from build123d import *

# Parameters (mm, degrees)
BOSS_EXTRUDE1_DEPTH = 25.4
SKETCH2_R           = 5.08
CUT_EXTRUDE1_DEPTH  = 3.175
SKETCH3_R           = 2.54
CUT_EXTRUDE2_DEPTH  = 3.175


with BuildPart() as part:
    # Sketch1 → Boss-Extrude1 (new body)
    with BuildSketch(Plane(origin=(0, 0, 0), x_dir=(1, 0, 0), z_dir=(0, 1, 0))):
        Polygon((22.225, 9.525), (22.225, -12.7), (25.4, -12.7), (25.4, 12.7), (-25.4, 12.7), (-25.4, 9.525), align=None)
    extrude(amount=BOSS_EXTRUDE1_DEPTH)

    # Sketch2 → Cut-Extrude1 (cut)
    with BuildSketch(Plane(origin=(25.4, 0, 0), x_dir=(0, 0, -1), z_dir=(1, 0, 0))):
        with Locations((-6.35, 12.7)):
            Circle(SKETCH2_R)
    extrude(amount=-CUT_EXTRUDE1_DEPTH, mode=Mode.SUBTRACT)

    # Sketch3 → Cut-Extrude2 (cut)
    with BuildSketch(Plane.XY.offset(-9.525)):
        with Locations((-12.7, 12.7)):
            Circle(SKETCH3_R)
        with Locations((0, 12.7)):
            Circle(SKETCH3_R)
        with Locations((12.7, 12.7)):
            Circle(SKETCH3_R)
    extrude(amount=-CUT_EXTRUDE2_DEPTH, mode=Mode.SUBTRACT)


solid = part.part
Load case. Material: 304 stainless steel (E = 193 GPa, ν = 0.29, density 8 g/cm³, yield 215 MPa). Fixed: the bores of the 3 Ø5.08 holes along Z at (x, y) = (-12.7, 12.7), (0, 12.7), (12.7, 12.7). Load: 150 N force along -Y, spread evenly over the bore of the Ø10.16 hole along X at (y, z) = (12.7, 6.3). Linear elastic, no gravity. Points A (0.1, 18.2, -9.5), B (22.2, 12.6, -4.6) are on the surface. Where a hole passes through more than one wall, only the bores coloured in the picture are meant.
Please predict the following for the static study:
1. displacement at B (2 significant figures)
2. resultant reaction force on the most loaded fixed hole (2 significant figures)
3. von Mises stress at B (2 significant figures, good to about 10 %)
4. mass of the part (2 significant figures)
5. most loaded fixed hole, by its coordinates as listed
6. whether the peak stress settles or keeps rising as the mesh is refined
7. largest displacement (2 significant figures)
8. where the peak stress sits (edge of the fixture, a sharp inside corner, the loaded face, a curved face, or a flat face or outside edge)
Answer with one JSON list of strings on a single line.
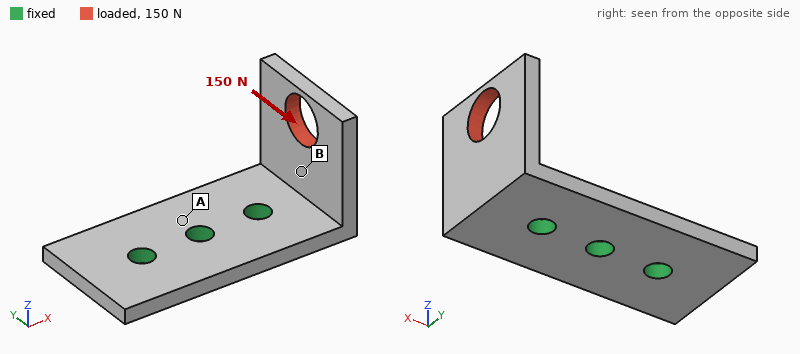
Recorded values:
["7.8 µm", "200 N", "16 MPa", "44 g", "(12.7, 12.7)", "keeps rising", "31 µm", "edge of the fixture"]
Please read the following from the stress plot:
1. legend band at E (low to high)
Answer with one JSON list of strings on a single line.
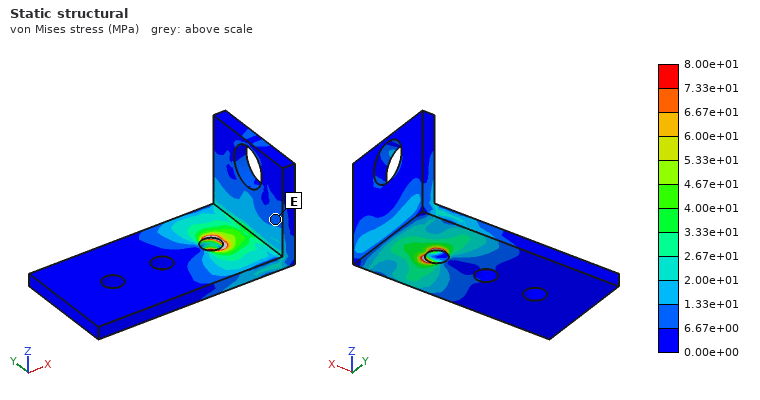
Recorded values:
["6.67e+00 to 1.33e+01 MPa"]
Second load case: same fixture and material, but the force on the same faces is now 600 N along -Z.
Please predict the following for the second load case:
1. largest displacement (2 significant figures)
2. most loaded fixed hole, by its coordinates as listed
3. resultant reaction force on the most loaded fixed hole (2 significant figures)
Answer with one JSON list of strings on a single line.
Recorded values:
["67 µm", "(12.7, 12.7)", "720 N"]
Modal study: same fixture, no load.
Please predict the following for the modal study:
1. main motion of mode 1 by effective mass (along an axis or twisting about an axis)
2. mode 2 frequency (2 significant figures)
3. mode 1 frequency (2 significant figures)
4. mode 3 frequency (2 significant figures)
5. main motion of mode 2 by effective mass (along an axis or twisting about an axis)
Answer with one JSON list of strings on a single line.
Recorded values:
["along X", "4300 Hz", "3000 Hz", "8300 Hz", "along Y"]
